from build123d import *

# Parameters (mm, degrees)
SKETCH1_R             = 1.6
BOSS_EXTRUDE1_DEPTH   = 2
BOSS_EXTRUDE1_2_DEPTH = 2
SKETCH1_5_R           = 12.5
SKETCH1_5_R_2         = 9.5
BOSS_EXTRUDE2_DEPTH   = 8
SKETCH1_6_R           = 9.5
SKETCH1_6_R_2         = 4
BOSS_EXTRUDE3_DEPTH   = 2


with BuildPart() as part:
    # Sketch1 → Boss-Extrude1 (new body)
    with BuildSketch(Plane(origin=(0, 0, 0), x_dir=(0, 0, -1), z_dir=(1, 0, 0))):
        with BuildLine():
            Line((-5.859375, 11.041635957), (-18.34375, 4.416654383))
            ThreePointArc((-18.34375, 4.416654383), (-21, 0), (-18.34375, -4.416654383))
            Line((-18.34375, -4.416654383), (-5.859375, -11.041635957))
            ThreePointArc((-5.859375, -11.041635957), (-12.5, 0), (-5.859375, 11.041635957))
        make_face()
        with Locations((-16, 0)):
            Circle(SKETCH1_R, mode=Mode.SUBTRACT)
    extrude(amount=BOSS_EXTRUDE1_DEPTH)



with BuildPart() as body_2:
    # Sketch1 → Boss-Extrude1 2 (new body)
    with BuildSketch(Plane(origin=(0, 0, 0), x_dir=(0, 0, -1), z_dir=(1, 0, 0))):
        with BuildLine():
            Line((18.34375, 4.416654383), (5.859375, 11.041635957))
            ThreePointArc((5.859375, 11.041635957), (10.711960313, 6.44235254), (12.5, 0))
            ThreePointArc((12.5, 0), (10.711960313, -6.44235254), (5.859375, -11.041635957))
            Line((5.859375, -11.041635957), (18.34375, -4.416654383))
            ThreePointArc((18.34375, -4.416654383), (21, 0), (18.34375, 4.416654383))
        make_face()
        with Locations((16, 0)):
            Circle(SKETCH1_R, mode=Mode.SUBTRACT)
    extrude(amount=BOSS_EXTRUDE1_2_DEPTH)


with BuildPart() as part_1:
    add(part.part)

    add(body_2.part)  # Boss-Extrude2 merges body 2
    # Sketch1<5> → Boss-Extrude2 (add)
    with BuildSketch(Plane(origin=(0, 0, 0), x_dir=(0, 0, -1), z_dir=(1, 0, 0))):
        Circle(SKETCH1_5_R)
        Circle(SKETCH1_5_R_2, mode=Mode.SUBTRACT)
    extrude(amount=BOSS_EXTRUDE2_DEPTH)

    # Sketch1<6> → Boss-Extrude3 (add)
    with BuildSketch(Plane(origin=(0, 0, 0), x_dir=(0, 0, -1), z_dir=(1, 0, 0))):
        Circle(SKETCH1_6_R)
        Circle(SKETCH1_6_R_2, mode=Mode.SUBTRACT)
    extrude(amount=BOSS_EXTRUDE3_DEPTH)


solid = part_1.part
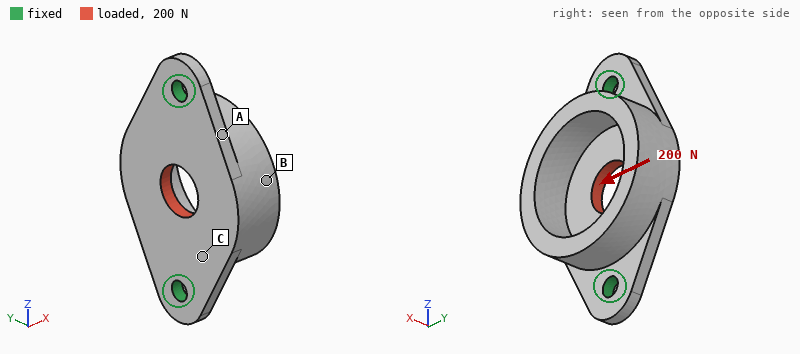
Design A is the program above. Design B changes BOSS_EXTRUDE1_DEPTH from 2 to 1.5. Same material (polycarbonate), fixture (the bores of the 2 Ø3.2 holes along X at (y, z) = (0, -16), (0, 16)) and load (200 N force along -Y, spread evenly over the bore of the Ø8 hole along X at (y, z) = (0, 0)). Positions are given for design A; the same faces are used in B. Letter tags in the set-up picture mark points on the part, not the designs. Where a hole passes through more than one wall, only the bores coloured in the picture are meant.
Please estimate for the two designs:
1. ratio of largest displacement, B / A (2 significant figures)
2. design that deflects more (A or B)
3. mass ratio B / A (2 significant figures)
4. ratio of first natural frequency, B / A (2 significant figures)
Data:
1.1
B
0.98
0.87
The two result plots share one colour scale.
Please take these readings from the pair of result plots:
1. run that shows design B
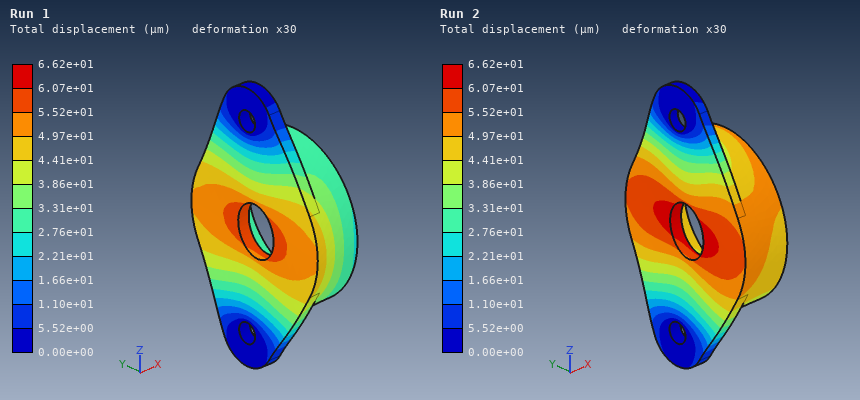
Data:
Run 2
